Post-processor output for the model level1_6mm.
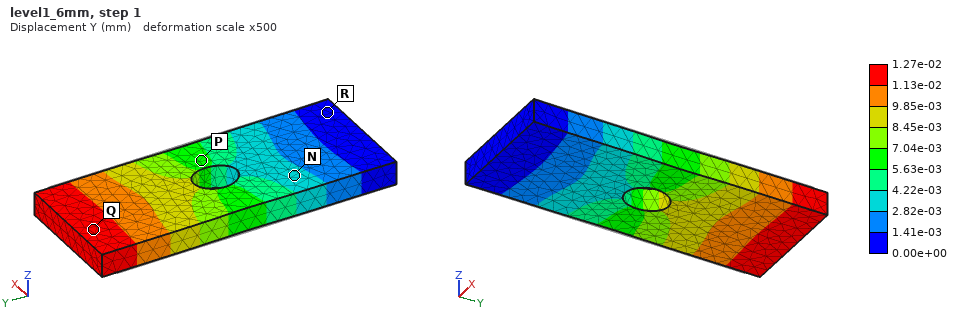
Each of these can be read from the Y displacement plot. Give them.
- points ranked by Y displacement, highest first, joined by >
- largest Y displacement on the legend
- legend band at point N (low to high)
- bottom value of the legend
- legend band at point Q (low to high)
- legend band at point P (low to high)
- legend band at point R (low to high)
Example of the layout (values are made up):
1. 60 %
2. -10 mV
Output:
1. Q > P > N > R
2. 1.27e-02 mm
3. 2.82e-03 to 4.22e-03 mm
4. 0.00e+00 mm
5. 1.13e-02 to 1.27e-02 mm
6. 5.63e-03 to 7.04e-03 mm
7. 0.00e+00 to 1.41e-03 mm
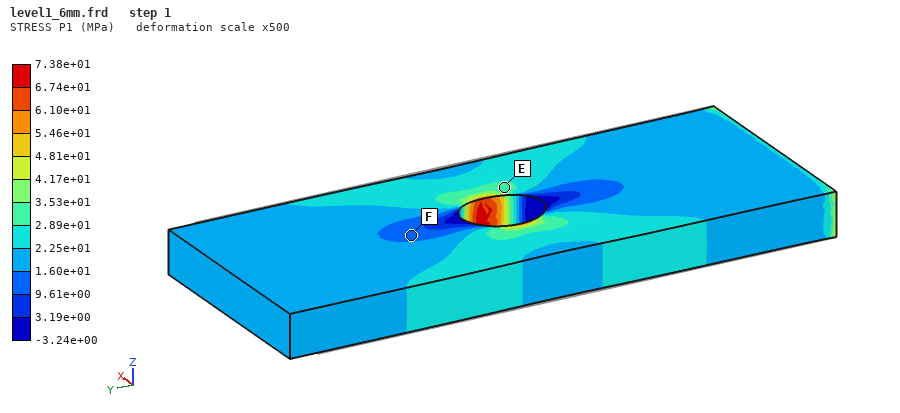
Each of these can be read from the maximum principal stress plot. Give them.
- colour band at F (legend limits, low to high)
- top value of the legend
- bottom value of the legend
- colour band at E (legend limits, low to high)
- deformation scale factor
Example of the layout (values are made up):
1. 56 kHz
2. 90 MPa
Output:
1. 9.61e+00 to 1.60e+01 MPa
2. 7.38e+01 MPa
3. -3.24e+00 MPa
4. 2.89e+01 to 3.53e+01 MPa
5. 500
